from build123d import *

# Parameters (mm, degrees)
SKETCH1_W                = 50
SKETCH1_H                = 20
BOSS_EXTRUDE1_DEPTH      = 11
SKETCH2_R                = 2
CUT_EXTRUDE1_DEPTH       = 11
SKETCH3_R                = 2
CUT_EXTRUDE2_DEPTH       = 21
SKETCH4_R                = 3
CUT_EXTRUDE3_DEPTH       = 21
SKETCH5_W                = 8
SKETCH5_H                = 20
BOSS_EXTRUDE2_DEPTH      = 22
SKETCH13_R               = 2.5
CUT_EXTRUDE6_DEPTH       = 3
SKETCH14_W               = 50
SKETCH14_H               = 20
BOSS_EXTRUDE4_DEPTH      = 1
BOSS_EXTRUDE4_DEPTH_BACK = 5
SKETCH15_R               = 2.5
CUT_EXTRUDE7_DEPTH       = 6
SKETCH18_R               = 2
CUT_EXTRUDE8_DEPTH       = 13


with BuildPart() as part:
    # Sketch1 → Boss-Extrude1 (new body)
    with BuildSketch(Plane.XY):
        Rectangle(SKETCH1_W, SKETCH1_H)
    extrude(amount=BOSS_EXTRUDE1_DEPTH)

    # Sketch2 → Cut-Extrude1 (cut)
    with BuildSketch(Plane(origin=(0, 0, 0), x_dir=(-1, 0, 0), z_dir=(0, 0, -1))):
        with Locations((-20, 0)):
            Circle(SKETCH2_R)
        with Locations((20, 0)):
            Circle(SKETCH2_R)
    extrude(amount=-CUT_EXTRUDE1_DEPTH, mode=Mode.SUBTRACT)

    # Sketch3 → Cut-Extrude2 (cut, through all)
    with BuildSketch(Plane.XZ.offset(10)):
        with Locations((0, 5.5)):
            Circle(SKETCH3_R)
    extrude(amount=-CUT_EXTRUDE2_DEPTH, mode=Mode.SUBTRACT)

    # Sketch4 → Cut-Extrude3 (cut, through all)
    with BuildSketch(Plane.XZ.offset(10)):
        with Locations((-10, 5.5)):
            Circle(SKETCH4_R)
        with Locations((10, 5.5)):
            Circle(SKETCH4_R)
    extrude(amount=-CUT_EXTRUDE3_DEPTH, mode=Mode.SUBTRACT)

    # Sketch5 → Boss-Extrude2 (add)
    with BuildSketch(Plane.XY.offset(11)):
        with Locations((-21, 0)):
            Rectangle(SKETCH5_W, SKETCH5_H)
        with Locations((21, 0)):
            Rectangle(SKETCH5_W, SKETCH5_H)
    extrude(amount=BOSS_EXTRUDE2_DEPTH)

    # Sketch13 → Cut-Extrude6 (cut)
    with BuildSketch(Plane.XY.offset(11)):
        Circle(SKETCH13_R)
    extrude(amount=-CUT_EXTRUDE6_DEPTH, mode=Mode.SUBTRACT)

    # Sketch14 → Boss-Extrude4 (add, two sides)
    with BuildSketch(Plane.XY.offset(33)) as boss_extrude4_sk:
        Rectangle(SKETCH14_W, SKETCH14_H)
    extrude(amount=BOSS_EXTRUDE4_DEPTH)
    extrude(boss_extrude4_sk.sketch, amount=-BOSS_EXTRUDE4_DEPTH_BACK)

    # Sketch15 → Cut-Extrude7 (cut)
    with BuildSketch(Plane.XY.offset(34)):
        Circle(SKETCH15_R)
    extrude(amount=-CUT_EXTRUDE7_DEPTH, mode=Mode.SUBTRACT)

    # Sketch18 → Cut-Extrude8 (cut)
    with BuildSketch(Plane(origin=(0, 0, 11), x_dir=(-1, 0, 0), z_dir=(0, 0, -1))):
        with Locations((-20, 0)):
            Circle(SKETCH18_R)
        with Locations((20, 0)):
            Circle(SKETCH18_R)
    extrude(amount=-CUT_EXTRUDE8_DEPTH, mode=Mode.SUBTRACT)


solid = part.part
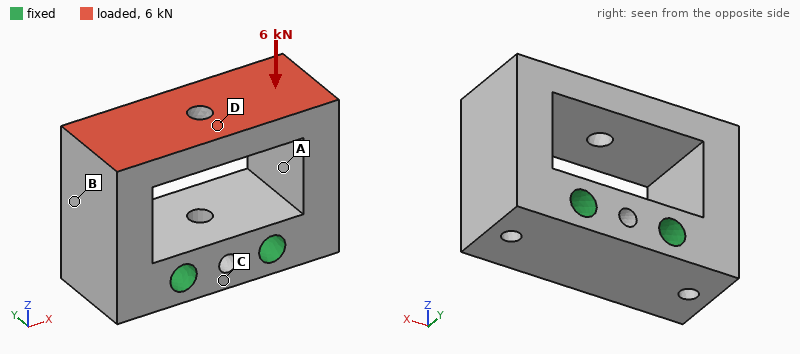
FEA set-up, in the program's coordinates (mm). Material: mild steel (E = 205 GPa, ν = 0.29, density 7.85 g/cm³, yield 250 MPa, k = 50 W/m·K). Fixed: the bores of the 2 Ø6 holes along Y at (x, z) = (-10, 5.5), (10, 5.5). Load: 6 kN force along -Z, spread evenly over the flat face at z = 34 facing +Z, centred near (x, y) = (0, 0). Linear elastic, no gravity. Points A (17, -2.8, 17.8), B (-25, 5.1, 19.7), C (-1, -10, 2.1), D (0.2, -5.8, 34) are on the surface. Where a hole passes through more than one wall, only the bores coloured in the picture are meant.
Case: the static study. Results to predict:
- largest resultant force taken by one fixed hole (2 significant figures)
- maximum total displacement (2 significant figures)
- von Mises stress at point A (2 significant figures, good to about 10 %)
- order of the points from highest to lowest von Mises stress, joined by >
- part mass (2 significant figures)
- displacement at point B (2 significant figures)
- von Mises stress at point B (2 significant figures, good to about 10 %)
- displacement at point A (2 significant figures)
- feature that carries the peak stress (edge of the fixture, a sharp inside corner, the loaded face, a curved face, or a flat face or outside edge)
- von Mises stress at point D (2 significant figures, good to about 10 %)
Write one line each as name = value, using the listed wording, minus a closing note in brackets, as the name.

largest resultant force taken by one fixed hole = 3.0 kN
maximum total displacement = 27 µm
von Mises stress at point A = 66 MPa
order of the points from highest to lowest von Mises stress, joined by > = D > A > B > C
part mass = 160 g
displacement at point B = 6.7 µm
von Mises stress at point B = 26 MPa
displacement at point A = 6.1 µm
feature that carries the peak stress = the loaded face
von Mises stress at point D = 93 MPa
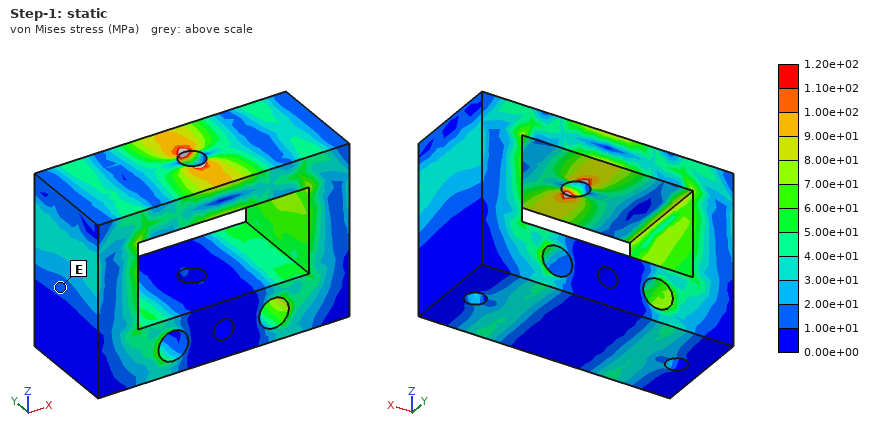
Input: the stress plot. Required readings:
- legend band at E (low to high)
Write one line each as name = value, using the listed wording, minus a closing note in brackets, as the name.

legend band at E = 1.00e+01 to 2.00e+01 MPa
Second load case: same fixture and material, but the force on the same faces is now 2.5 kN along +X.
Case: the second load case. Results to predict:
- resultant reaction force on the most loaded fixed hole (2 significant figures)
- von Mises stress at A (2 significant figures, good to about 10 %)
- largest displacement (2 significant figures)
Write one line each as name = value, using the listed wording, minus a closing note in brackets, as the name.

resultant reaction force on the most loaded fixed hole = 1.6 kN
von Mises stress at A = 19 MPa
largest displacement = 34 µm
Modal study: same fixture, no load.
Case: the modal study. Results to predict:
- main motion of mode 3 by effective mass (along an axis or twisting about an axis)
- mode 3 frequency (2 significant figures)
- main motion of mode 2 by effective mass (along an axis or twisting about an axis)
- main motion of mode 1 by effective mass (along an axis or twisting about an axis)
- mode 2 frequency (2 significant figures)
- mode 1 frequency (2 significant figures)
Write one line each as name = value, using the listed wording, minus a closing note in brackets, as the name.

main motion of mode 3 by effective mass = twisting about Z
mode 3 frequency = 11 kHz
main motion of mode 2 by effective mass = along Y
main motion of mode 1 by effective mass = along X
mode 2 frequency = 7100 Hz
mode 1 frequency = 6000 Hz
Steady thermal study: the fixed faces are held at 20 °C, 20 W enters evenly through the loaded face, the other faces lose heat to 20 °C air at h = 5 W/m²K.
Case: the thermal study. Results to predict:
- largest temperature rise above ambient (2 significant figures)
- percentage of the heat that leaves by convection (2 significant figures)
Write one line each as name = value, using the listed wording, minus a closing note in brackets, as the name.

largest temperature rise above ambient = 48 K
percentage of the heat that leaves by convection = 3.1 %
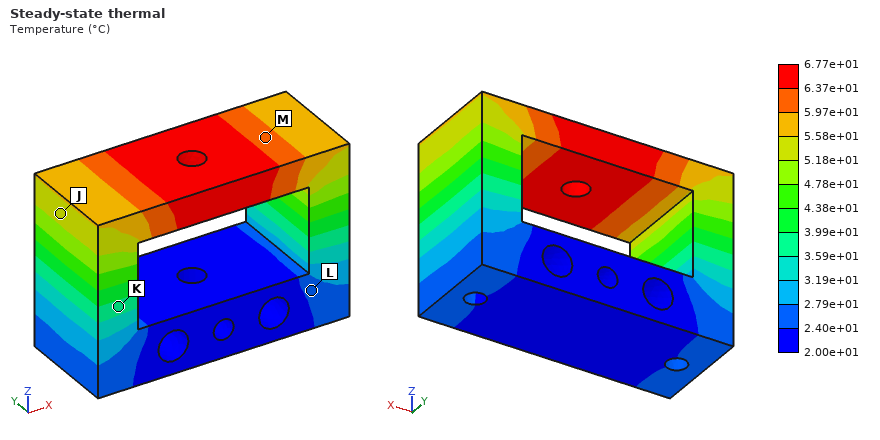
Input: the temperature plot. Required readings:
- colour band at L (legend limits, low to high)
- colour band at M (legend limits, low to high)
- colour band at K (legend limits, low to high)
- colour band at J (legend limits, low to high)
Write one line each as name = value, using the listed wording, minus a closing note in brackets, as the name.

colour band at L = 2.40e+01 to 2.79e+01 °C
colour band at M = 5.97e+01 to 6.37e+01 °C
colour band at K = 3.59e+01 to 3.99e+01 °C
colour band at J = 5.18e+01 to 5.58e+01 °C
